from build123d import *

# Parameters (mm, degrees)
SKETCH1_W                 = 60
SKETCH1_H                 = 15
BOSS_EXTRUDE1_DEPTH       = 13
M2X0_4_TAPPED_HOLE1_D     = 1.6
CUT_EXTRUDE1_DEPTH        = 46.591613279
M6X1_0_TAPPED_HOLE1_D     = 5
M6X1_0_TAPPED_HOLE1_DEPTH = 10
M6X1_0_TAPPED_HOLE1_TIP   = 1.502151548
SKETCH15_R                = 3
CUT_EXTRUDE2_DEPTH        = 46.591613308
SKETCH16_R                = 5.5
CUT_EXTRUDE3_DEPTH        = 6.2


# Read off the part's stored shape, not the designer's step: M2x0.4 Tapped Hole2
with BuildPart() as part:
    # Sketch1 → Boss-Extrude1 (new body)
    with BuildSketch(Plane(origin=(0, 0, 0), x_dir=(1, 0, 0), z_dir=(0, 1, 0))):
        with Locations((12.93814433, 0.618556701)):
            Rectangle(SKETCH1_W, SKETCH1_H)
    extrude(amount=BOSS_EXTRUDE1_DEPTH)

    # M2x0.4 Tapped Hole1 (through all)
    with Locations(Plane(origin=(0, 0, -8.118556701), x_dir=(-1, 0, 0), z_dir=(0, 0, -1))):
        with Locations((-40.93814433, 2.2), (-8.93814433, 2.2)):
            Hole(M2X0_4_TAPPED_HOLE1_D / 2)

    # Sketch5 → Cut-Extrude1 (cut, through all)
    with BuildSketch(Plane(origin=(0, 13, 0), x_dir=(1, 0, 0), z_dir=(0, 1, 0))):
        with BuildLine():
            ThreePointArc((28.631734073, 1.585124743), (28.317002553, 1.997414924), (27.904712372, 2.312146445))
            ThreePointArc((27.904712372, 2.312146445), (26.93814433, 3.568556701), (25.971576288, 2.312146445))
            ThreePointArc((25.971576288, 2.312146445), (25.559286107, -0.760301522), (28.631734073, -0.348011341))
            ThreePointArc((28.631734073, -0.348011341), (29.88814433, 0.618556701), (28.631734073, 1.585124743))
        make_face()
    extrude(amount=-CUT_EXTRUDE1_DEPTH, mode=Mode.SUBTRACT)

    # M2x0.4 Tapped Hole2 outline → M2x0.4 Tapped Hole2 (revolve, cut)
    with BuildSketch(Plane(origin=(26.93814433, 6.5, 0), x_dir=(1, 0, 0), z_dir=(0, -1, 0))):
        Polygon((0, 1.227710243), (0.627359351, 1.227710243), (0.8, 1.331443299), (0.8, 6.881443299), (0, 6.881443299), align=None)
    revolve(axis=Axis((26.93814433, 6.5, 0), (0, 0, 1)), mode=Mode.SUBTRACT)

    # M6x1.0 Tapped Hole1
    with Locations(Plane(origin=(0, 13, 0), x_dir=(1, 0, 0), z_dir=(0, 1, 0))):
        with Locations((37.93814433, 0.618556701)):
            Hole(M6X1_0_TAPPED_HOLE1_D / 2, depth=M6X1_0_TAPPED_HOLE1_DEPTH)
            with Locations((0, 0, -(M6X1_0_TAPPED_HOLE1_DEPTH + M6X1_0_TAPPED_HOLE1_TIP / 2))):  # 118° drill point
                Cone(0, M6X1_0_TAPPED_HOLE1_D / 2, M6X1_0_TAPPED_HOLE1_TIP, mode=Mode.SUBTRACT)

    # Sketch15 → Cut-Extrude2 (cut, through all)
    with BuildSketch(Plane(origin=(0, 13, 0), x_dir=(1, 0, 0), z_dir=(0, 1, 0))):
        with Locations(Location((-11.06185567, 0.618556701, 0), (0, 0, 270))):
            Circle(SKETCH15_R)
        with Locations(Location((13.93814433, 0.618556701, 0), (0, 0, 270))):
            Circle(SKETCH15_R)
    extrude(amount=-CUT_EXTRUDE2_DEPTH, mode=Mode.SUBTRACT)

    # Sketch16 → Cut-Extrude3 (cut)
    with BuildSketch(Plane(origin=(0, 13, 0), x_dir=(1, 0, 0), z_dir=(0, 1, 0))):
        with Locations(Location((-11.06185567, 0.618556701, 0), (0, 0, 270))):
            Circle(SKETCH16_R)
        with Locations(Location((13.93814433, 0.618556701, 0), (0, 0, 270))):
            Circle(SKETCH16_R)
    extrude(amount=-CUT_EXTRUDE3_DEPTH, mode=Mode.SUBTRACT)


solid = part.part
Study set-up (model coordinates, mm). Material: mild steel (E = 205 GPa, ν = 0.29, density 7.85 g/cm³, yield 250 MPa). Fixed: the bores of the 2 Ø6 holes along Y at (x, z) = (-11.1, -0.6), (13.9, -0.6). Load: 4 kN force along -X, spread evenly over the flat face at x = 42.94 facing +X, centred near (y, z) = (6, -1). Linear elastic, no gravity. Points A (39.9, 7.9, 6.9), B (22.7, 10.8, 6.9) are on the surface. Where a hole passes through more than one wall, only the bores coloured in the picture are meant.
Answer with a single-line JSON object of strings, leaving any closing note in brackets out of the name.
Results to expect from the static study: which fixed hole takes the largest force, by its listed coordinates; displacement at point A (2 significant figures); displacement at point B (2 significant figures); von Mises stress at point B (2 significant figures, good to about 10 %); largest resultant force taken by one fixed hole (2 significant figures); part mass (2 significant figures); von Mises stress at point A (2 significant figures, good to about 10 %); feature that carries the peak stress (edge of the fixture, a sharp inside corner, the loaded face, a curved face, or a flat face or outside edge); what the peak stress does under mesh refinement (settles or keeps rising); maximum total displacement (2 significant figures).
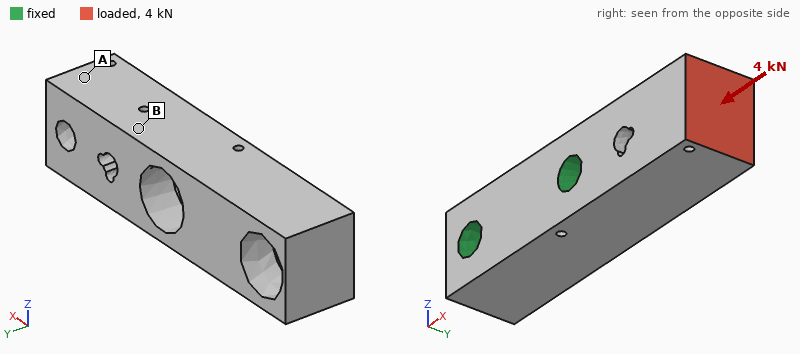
{"which fixed hole takes the largest force, by its listed coordinates": "(13.9, -0.6)", "displacement at point A": "8.3 µm", "displacement at point B": "3.9 µm", "von Mises stress at point B": "35 MPa", "largest resultant force taken by one fixed hole": "3.4 kN", "part mass": "76 g", "von Mises stress at point A": "15 MPa", "feature that carries the peak stress": "a sharp inside corner", "what the peak stress does under mesh refinement": "keeps rising", "maximum total displacement": "11 µm"}
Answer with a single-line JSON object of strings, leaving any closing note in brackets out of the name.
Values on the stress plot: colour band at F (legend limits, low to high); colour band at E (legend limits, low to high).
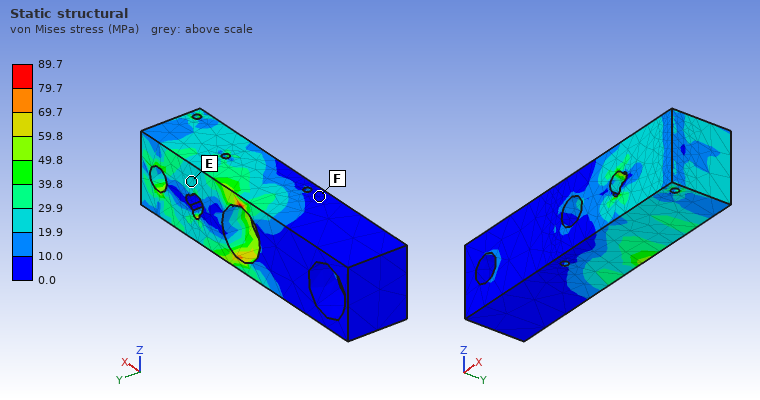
{"colour band at F": "0.0 to 10.0 MPa", "colour band at E": "19.9 to 29.9 MPa"}
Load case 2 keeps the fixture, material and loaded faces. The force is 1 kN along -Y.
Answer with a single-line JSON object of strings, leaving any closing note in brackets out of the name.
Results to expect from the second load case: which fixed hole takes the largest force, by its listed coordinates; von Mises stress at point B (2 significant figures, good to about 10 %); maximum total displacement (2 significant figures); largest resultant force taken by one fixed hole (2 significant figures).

{"which fixed hole takes the largest force, by its listed coordinates": "(13.9, -0.6)", "von Mises stress at point B": "55 MPa", "maximum total displacement": "33 µm", "largest resultant force taken by one fixed hole": "1.7 kN"}
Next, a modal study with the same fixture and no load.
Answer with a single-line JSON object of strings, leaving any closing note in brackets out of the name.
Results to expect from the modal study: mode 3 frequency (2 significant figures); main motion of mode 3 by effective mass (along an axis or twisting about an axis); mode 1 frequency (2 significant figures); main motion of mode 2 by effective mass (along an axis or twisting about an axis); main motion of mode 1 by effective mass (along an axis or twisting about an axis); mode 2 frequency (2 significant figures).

{"mode 3 frequency": "19 kHz", "main motion of mode 3 by effective mass": "twisting about X", "mode 1 frequency": "8500 Hz", "main motion of mode 2 by effective mass": "along Z", "main motion of mode 1 by effective mass": "along Y", "mode 2 frequency": "10 kHz"}
